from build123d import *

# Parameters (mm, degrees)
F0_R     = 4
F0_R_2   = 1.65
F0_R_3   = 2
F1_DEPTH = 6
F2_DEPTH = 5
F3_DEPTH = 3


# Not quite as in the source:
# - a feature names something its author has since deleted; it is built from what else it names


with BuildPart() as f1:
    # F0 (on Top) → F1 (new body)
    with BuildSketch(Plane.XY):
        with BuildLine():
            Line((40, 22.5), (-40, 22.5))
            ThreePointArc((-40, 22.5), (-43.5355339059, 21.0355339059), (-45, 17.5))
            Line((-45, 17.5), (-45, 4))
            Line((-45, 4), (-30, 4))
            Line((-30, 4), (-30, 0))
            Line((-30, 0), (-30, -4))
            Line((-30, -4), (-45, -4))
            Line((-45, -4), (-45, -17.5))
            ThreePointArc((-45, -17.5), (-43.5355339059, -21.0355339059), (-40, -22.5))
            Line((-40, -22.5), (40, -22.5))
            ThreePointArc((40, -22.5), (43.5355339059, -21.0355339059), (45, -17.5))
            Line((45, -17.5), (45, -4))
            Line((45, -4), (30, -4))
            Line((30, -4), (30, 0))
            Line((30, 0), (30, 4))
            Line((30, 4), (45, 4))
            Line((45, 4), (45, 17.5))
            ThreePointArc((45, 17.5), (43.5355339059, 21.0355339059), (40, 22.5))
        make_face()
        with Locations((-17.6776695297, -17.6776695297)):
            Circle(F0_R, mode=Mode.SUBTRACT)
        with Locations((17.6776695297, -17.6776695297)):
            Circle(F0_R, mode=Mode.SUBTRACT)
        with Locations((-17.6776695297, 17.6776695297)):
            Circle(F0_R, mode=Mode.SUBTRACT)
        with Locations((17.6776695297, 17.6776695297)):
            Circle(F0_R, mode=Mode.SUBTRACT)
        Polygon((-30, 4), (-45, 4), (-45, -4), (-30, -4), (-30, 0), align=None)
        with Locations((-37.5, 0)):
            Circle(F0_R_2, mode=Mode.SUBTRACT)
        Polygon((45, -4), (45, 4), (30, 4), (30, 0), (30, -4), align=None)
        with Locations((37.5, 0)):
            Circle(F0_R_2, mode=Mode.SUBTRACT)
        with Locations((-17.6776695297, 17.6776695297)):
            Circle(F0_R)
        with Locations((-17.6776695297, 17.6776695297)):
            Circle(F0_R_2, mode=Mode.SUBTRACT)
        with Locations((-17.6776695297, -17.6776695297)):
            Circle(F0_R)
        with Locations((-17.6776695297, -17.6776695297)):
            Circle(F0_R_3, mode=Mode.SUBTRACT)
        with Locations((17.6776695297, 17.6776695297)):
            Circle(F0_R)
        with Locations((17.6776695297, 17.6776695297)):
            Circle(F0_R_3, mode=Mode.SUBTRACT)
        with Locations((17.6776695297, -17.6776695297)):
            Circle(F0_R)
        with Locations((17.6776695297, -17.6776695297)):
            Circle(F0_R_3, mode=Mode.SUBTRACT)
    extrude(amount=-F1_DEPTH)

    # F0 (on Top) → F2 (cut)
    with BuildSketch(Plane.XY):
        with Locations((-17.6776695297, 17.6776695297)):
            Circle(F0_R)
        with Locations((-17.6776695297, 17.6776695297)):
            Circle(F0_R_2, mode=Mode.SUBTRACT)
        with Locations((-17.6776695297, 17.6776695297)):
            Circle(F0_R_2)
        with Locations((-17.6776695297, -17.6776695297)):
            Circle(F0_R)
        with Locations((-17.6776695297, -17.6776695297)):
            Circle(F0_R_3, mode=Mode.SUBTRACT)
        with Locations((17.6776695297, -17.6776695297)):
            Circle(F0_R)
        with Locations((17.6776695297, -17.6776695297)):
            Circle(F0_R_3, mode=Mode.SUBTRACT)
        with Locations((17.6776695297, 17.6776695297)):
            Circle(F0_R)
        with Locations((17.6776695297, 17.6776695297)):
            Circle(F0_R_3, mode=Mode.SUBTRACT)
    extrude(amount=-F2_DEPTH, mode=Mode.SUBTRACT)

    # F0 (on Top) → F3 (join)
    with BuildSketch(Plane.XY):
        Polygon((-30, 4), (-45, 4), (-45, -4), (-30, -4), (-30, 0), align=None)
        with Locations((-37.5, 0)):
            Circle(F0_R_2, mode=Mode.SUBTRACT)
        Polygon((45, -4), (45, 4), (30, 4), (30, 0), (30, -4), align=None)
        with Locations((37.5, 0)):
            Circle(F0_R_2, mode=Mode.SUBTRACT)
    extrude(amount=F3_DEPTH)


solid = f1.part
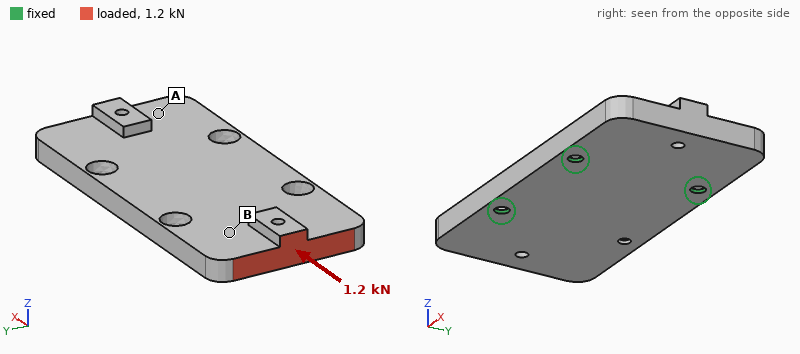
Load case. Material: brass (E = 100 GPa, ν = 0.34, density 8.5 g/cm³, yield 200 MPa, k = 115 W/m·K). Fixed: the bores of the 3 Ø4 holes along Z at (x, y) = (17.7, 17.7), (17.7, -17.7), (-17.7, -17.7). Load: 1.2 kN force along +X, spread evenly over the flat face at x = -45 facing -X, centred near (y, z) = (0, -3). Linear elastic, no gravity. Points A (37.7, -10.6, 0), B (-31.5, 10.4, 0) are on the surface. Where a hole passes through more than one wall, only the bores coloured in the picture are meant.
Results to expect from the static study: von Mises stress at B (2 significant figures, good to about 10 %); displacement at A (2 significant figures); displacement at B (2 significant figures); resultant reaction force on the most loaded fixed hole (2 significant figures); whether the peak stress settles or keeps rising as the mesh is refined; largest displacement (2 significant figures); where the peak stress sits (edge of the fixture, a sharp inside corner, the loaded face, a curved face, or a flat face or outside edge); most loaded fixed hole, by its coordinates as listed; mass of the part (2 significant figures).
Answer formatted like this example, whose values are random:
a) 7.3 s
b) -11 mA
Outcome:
a) 7.0 MPa
b) 6.9 µm
c) 14 µm
d) 480 N
e) keeps rising
f) 21 µm
g) edge of the fixture
h) (-17.7, -17.7)
i) 200 g
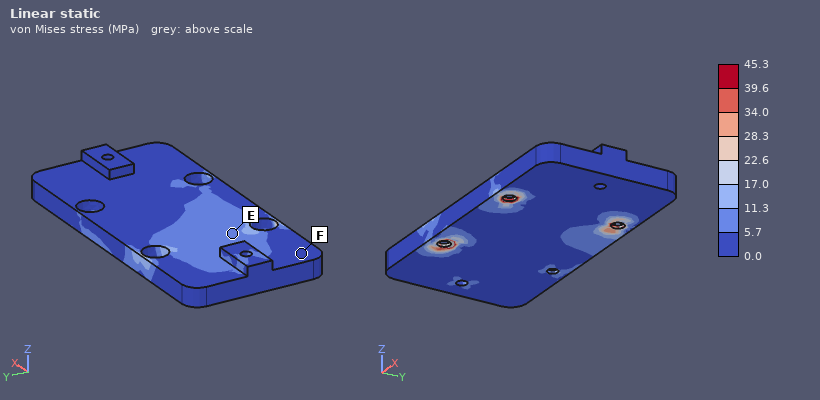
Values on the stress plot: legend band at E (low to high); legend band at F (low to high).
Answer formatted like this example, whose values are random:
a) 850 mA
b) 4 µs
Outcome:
a) 5.7 to 11.3 MPa
b) 0.0 to 5.7 MPa
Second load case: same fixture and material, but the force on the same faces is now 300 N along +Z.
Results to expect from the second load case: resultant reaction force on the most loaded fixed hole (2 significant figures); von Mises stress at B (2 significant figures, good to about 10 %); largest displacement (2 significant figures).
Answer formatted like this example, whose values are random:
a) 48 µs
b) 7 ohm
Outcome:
a) 640 N
b) 15 MPa
c) 0.16 mm
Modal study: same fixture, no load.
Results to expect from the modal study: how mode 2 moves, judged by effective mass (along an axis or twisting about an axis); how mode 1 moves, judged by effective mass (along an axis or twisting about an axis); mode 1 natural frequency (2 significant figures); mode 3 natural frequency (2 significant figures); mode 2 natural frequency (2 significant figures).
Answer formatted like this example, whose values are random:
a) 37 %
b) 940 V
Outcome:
a) along Z
b) along Z
c) 1300 Hz
d) 3600 Hz
e) 2400 Hz
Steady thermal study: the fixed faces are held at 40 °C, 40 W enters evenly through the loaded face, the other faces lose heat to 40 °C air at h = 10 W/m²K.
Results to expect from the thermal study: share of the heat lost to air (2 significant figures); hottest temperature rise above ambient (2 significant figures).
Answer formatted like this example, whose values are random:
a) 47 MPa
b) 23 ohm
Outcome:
a) 7.0 %
b) 74 K
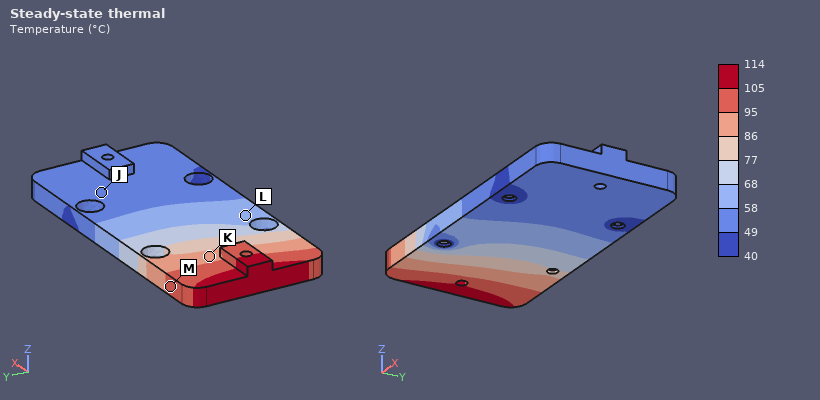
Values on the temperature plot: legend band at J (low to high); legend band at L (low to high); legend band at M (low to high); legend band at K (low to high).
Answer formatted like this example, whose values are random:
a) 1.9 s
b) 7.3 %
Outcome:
a) 49 to 58 °C
b) 58 to 68 °C
c) 95 to 105 °C
d) 86 to 95 °C
